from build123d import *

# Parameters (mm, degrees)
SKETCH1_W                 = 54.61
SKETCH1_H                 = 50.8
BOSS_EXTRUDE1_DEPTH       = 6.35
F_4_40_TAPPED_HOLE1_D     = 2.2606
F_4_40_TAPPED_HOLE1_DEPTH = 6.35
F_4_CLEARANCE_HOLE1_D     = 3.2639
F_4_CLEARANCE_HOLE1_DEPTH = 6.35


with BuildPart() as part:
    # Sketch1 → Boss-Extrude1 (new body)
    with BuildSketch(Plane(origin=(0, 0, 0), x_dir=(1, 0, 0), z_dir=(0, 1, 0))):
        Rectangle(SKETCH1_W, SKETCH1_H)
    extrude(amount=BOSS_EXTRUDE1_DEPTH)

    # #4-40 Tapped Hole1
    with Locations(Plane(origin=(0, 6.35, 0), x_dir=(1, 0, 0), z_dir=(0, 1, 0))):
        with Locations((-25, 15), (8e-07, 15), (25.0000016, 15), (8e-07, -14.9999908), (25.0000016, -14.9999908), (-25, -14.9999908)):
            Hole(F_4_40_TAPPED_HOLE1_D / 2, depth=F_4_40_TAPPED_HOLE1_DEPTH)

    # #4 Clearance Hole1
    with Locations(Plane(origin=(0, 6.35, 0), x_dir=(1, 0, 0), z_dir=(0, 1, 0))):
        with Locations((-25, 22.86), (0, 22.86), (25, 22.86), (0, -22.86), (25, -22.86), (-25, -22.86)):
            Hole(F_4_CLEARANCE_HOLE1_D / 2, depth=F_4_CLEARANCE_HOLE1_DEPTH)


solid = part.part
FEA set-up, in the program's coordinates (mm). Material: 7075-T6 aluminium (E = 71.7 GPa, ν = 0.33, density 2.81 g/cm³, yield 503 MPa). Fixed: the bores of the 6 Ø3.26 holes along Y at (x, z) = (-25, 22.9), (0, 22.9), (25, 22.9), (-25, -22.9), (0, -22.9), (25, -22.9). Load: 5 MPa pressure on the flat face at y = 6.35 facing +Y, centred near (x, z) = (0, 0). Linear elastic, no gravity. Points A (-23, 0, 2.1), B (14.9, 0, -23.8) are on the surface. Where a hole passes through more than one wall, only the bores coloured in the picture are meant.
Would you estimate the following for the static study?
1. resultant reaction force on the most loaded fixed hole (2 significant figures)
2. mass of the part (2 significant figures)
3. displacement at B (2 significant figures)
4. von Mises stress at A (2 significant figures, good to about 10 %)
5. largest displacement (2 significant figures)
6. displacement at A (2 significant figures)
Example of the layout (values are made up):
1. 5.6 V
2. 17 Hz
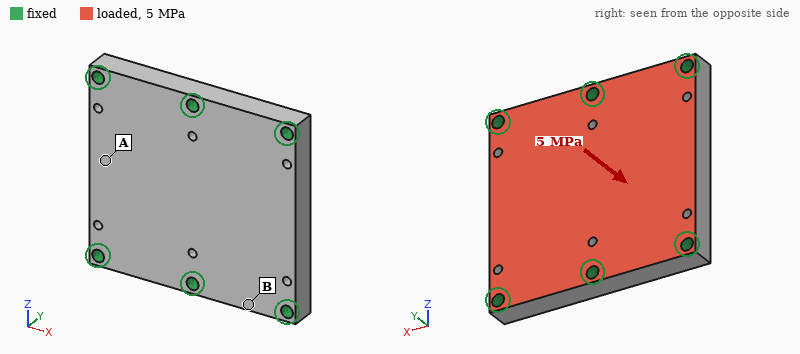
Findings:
1. 3.1 kN
2. 48 g
3. 10.0 µm
4. 78 MPa
5. 64 µm
6. 61 µm
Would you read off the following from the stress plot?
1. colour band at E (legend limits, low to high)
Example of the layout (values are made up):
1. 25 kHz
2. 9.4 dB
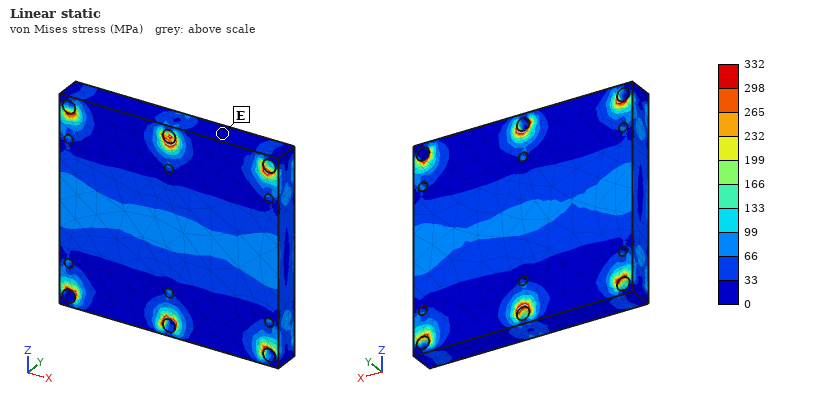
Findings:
1. 0 to 33 MPa
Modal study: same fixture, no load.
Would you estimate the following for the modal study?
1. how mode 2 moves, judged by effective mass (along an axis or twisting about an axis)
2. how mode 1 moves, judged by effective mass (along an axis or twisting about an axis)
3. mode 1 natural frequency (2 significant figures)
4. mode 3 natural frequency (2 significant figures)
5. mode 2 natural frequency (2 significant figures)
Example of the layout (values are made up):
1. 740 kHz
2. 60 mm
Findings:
1. twisting about Z
2. along Y
3. 12 kHz
4. 22 kHz
5. 14 kHz
